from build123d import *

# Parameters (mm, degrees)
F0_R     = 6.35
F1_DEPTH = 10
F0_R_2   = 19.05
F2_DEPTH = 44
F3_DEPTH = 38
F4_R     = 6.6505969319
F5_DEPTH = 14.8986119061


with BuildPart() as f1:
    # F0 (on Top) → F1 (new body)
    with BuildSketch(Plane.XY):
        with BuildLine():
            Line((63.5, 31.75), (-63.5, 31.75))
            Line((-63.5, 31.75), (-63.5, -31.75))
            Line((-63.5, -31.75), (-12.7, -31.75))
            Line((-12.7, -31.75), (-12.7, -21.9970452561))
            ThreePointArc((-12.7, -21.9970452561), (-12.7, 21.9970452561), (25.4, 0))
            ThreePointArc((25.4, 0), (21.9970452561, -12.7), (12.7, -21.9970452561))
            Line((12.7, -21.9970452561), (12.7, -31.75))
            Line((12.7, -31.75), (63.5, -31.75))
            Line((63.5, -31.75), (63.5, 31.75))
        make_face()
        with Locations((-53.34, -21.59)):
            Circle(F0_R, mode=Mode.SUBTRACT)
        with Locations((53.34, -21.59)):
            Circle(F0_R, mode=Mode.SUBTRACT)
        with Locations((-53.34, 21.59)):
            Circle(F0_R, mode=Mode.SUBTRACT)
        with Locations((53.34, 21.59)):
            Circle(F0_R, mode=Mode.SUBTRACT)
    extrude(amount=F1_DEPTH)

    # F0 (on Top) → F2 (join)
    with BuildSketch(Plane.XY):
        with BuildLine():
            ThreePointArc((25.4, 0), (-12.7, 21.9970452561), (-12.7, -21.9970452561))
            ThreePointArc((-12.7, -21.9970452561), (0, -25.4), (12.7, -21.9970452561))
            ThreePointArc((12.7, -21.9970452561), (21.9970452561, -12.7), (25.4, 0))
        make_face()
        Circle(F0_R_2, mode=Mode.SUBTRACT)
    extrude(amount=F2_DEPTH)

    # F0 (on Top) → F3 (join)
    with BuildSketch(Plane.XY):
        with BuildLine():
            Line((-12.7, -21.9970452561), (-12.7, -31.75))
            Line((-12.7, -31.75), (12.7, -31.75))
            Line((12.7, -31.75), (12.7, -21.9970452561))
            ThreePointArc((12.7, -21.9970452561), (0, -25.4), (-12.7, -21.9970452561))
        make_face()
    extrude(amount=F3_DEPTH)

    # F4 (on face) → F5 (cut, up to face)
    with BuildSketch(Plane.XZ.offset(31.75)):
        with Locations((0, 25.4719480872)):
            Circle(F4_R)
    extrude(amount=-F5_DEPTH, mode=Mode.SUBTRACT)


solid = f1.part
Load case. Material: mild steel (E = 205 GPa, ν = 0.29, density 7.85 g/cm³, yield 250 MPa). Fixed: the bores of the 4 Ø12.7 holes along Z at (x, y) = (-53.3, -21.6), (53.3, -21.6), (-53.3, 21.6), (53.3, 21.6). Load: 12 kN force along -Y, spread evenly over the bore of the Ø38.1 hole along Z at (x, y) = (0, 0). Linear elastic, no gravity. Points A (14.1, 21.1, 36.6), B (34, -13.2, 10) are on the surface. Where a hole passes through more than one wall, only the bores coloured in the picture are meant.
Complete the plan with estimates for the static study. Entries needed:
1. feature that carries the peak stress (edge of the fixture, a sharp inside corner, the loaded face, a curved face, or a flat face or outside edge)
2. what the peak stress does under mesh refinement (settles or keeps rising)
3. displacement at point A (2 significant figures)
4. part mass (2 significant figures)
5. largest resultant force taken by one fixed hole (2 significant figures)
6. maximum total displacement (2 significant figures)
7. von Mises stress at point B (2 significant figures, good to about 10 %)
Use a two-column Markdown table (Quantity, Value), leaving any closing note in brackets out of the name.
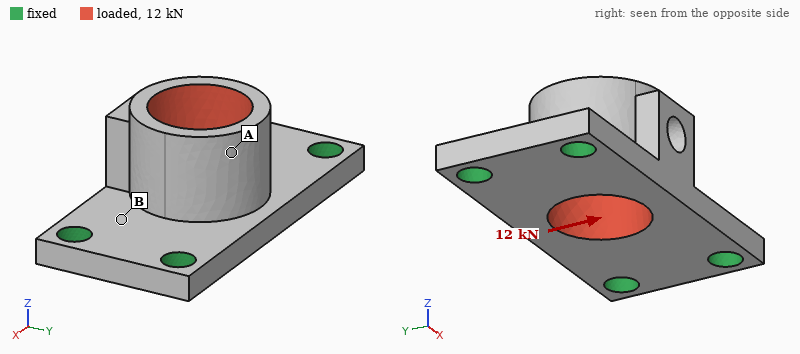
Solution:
| Quantity | Value |
|---|---|
| feature that carries the peak stress | edge of the fixture |
| what the peak stress does under mesh refinement | keeps rising |
| displacement at point A | 48 µm |
| part mass | 770 g |
| largest resultant force taken by one fixed hole | 4.8 kN |
| maximum total displacement | 59 µm |
| von Mises stress at point B | 62 MPa |
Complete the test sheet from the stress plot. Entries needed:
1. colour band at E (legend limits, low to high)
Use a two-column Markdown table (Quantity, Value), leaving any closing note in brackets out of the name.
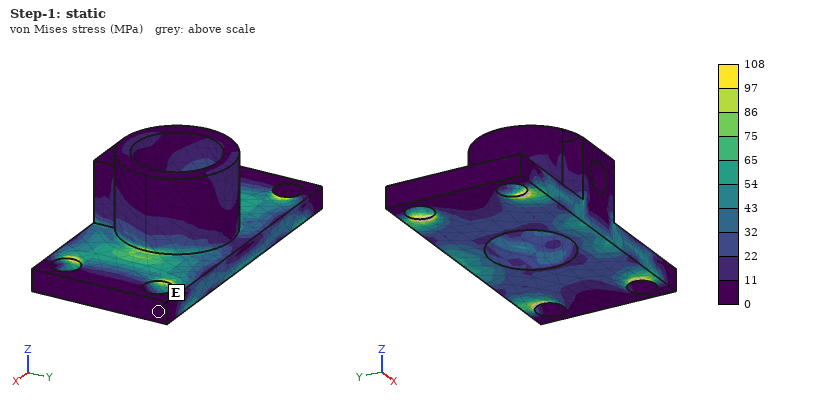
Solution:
| Quantity | Value |
|---|---|
| colour band at E | 0 to 11 MPa |
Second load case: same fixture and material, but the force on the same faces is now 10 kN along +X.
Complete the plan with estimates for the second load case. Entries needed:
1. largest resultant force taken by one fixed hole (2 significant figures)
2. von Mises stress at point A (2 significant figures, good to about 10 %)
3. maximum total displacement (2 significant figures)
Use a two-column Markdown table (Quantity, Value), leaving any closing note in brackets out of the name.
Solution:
| Quantity | Value |
|---|---|
| largest resultant force taken by one fixed hole | 2.8 kN |
| von Mises stress at point A | 6.2 MPa |
| maximum total displacement | 19 µm |
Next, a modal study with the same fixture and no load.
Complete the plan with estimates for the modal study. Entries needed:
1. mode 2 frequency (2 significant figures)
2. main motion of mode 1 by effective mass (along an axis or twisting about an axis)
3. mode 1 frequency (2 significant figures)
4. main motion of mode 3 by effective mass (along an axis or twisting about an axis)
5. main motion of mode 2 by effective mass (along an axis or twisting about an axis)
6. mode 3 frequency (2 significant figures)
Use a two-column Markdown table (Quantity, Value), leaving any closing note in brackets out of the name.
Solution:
| Quantity | Value |
|---|---|
| mode 2 frequency | 4600 Hz |
| main motion of mode 1 by effective mass | along Y |
| mode 1 frequency | 3900 Hz |
| main motion of mode 3 by effective mass | along X |
| main motion of mode 2 by effective mass | along Z |
| mode 3 frequency | 6500 Hz |
